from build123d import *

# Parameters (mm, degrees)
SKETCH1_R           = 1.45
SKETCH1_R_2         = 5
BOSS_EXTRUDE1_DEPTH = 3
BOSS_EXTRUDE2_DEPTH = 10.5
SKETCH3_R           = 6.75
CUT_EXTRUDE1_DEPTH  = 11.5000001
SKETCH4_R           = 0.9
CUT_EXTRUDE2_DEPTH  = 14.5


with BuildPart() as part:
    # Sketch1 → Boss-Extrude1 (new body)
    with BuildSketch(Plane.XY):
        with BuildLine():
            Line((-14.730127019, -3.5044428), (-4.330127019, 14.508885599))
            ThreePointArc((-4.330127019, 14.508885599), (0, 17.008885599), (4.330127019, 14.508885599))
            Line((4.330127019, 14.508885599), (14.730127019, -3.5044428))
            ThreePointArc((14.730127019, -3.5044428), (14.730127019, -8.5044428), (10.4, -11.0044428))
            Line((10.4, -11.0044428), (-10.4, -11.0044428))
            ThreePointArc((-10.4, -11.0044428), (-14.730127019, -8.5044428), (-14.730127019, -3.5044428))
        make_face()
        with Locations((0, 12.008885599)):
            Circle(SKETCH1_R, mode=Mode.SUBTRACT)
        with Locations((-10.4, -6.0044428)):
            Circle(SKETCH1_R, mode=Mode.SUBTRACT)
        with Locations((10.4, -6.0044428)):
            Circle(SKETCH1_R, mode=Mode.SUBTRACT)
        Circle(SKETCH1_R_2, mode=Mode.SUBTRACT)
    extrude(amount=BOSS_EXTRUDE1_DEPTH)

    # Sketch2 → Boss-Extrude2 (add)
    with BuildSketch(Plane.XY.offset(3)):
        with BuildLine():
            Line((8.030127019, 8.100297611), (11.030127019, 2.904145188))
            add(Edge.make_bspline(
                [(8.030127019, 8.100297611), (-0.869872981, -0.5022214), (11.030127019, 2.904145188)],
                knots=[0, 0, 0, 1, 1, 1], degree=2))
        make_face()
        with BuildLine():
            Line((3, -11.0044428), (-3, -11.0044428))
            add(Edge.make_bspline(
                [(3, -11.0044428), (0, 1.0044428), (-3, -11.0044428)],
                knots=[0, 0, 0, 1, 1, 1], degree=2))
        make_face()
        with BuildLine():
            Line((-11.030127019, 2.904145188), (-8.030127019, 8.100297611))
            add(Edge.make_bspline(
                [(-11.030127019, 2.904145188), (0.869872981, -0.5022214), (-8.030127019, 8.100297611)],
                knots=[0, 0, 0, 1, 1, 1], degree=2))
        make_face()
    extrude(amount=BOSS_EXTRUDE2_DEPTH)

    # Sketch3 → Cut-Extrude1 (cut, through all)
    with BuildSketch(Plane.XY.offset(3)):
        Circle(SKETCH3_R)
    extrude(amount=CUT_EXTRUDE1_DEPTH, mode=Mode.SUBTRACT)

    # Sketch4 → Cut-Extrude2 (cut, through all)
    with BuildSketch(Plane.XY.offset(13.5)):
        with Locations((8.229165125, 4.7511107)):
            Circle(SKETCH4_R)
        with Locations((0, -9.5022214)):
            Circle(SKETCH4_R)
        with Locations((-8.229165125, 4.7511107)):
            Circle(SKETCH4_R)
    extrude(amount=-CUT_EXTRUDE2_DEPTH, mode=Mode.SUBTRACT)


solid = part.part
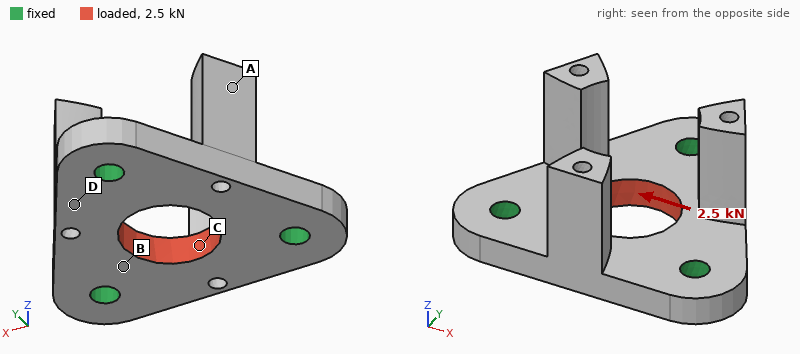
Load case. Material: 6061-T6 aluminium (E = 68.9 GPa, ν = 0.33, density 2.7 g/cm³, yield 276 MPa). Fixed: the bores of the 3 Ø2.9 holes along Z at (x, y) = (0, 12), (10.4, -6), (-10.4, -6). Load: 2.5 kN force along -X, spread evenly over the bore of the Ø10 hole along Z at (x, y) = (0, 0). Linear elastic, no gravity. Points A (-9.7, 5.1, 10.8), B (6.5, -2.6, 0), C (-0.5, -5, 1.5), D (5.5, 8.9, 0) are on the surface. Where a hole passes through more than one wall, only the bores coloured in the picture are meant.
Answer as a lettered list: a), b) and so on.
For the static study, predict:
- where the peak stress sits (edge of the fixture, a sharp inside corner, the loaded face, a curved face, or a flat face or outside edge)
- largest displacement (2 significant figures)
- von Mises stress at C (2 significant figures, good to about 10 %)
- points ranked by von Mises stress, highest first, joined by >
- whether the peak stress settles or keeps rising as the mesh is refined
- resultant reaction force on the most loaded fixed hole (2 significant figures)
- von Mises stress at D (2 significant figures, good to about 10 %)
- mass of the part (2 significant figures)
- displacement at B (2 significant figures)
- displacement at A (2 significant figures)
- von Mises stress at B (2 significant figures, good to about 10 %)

a) edge of the fixture
b) 12 µm
c) 46 MPa
d) C > B > D > A
e) keeps rising
f) 860 N
g) 25 MPa
h) 5.3 g
i) 4.4 µm
j) 12 µm
k) 37 MPa
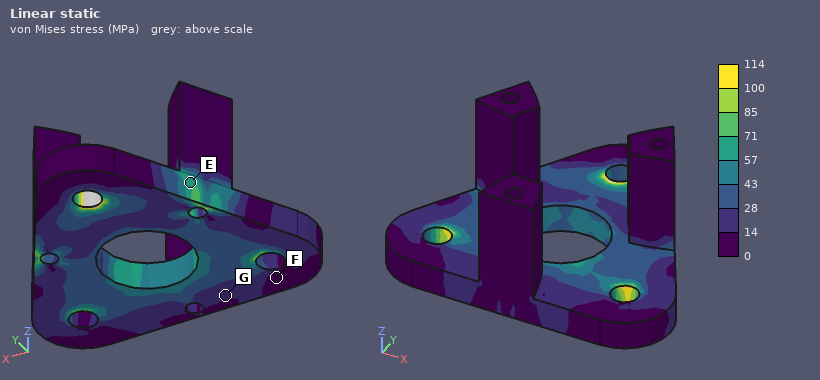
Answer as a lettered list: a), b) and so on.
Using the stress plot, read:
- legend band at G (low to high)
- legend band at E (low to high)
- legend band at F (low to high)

a) 14 to 28 MPa
b) 57 to 71 MPa
c) 0 to 14 MPa
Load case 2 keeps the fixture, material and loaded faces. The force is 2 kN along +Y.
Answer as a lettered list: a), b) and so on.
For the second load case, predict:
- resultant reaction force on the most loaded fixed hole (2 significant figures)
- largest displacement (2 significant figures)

a) 700 N
b) 11 µm
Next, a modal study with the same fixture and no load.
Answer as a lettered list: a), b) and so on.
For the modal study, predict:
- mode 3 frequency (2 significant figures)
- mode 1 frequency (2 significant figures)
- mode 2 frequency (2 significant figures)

a) 14 kHz
b) 14 kHz
c) 14 kHz
